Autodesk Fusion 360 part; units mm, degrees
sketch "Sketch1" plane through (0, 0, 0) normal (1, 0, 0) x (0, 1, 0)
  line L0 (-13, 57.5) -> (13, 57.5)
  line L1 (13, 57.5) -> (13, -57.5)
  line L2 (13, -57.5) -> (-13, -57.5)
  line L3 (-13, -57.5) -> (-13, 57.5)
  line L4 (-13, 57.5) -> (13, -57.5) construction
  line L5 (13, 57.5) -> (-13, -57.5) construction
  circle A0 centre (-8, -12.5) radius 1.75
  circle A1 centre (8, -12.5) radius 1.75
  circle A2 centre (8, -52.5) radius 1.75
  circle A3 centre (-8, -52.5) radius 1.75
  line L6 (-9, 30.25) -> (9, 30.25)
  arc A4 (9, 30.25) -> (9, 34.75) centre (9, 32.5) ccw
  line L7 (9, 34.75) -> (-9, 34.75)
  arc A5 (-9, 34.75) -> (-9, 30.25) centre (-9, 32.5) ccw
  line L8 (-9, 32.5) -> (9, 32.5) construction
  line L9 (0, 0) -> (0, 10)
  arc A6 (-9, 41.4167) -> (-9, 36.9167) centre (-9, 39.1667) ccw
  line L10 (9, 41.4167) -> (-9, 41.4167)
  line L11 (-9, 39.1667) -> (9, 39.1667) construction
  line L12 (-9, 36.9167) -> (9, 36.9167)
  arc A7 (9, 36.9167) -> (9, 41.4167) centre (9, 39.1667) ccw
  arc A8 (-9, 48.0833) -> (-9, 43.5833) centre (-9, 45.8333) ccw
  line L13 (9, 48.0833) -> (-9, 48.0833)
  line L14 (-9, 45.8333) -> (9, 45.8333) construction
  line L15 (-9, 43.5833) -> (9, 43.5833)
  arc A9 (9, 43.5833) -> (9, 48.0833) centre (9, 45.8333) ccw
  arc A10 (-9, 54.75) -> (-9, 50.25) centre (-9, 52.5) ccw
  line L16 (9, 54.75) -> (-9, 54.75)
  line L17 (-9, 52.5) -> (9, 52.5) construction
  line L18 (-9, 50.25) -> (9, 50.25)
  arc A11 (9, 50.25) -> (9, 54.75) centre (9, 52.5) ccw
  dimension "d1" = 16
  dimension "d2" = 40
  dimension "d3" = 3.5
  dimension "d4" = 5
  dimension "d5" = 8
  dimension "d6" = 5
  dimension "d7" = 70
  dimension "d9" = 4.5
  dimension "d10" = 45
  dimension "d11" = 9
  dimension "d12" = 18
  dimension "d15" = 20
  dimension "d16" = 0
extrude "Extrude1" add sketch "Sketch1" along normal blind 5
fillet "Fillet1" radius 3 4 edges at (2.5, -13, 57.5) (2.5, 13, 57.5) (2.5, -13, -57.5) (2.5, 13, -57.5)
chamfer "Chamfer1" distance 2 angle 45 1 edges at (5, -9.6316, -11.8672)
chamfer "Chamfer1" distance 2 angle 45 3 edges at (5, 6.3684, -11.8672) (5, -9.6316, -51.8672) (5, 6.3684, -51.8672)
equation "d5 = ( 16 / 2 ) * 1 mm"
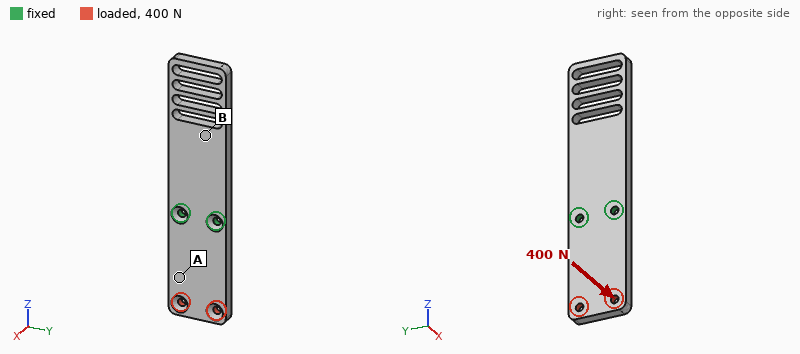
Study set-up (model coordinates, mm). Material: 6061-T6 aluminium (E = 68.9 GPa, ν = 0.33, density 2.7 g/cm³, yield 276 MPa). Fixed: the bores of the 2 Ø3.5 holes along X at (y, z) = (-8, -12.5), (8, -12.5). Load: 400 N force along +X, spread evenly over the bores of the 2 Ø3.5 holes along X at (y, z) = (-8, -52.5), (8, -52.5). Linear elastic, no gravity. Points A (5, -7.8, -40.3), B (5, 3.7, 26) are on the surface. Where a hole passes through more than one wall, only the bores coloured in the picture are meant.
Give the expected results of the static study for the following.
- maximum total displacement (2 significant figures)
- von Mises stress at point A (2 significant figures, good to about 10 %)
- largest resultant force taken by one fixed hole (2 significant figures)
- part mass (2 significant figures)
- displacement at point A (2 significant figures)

0.67 mm
46 MPa
260 N
34 g
0.33 mm
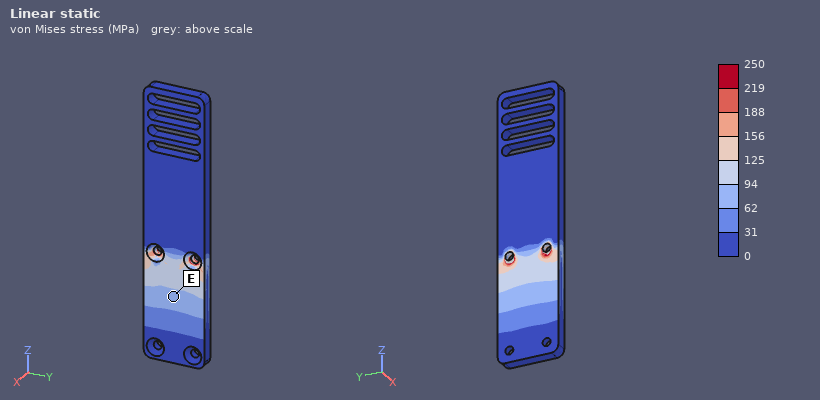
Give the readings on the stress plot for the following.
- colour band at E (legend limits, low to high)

62 to 94 MPa
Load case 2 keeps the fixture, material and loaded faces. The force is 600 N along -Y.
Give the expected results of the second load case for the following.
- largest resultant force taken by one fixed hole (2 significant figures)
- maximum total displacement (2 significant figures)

1.4 kN
51 µm
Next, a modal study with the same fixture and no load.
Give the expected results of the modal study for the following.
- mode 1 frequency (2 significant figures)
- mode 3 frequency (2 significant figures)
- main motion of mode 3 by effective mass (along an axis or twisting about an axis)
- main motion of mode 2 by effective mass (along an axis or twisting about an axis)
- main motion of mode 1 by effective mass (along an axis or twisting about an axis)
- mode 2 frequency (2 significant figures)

980 Hz
3400 Hz
along Y
along X
along X
1900 Hz
